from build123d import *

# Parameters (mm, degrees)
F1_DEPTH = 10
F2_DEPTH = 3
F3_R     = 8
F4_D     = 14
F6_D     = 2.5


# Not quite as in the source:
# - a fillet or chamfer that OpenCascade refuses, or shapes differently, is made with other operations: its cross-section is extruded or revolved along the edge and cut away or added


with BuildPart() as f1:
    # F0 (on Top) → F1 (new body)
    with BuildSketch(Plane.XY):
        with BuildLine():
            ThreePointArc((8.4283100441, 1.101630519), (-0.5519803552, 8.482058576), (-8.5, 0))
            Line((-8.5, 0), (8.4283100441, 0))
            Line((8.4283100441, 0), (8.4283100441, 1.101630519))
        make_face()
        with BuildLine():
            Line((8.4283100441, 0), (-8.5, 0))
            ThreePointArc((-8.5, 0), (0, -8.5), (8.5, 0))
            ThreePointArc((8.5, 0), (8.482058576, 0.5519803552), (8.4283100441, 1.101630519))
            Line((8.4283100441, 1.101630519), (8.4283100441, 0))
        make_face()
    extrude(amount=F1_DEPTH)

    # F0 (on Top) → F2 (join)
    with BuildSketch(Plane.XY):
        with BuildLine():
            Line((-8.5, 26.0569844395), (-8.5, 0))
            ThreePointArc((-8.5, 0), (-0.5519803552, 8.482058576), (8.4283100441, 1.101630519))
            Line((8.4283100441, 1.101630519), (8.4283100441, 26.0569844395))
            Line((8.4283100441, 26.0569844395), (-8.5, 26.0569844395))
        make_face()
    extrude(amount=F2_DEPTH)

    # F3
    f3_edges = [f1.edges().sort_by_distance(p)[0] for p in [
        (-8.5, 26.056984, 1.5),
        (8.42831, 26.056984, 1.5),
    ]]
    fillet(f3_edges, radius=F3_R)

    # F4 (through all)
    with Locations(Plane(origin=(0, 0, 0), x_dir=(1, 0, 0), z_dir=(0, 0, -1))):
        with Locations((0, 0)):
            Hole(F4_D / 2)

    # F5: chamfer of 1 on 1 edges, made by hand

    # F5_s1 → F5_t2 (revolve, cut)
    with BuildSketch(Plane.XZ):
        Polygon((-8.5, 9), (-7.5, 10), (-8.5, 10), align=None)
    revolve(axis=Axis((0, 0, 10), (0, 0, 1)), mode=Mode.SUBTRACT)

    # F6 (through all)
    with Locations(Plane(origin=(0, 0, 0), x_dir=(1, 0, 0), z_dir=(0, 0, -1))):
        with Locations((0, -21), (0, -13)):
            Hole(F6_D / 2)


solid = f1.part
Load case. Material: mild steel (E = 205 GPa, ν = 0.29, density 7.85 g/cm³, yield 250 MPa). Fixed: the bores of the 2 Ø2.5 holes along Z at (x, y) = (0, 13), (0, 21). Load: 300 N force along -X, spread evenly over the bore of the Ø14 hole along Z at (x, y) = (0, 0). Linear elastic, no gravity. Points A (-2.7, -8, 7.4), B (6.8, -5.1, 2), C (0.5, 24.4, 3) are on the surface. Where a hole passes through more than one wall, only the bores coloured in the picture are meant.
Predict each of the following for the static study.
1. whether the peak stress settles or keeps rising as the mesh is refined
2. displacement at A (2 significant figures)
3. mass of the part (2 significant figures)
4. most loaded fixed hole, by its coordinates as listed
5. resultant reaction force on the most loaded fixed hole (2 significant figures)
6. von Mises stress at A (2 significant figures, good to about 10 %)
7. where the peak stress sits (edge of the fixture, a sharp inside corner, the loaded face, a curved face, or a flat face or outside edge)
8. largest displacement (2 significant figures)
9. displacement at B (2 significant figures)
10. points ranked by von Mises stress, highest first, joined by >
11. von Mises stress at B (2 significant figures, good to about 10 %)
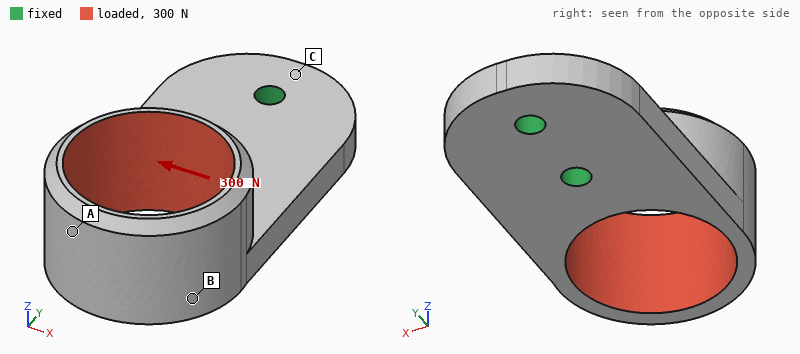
keeps rising
26 µm
12 g
(0, 13)
650 N
25 MPa
edge of the fixture
27 µm
22 µm
B > A > C
45 MPa
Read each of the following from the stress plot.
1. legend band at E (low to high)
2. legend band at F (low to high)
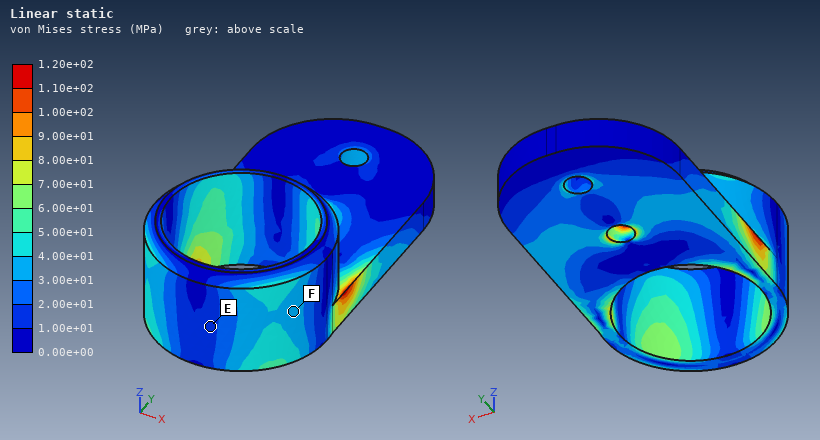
1.00e+01 to 2.00e+01 MPa
3.00e+01 to 4.00e+01 MPa
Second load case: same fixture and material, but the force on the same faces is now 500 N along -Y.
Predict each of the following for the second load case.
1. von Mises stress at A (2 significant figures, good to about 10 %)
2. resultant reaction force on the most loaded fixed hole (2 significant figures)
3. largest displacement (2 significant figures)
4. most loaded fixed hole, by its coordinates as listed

31 MPa
330 N
53 µm
(0, 13)
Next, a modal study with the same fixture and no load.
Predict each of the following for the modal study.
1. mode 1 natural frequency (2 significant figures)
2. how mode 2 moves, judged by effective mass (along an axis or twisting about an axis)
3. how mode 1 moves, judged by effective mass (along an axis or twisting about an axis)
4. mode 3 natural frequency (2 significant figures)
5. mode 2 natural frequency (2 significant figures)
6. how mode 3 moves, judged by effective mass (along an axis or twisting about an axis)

4800 Hz
along X
along Z
10 kHz
8100 Hz
twisting about Y
